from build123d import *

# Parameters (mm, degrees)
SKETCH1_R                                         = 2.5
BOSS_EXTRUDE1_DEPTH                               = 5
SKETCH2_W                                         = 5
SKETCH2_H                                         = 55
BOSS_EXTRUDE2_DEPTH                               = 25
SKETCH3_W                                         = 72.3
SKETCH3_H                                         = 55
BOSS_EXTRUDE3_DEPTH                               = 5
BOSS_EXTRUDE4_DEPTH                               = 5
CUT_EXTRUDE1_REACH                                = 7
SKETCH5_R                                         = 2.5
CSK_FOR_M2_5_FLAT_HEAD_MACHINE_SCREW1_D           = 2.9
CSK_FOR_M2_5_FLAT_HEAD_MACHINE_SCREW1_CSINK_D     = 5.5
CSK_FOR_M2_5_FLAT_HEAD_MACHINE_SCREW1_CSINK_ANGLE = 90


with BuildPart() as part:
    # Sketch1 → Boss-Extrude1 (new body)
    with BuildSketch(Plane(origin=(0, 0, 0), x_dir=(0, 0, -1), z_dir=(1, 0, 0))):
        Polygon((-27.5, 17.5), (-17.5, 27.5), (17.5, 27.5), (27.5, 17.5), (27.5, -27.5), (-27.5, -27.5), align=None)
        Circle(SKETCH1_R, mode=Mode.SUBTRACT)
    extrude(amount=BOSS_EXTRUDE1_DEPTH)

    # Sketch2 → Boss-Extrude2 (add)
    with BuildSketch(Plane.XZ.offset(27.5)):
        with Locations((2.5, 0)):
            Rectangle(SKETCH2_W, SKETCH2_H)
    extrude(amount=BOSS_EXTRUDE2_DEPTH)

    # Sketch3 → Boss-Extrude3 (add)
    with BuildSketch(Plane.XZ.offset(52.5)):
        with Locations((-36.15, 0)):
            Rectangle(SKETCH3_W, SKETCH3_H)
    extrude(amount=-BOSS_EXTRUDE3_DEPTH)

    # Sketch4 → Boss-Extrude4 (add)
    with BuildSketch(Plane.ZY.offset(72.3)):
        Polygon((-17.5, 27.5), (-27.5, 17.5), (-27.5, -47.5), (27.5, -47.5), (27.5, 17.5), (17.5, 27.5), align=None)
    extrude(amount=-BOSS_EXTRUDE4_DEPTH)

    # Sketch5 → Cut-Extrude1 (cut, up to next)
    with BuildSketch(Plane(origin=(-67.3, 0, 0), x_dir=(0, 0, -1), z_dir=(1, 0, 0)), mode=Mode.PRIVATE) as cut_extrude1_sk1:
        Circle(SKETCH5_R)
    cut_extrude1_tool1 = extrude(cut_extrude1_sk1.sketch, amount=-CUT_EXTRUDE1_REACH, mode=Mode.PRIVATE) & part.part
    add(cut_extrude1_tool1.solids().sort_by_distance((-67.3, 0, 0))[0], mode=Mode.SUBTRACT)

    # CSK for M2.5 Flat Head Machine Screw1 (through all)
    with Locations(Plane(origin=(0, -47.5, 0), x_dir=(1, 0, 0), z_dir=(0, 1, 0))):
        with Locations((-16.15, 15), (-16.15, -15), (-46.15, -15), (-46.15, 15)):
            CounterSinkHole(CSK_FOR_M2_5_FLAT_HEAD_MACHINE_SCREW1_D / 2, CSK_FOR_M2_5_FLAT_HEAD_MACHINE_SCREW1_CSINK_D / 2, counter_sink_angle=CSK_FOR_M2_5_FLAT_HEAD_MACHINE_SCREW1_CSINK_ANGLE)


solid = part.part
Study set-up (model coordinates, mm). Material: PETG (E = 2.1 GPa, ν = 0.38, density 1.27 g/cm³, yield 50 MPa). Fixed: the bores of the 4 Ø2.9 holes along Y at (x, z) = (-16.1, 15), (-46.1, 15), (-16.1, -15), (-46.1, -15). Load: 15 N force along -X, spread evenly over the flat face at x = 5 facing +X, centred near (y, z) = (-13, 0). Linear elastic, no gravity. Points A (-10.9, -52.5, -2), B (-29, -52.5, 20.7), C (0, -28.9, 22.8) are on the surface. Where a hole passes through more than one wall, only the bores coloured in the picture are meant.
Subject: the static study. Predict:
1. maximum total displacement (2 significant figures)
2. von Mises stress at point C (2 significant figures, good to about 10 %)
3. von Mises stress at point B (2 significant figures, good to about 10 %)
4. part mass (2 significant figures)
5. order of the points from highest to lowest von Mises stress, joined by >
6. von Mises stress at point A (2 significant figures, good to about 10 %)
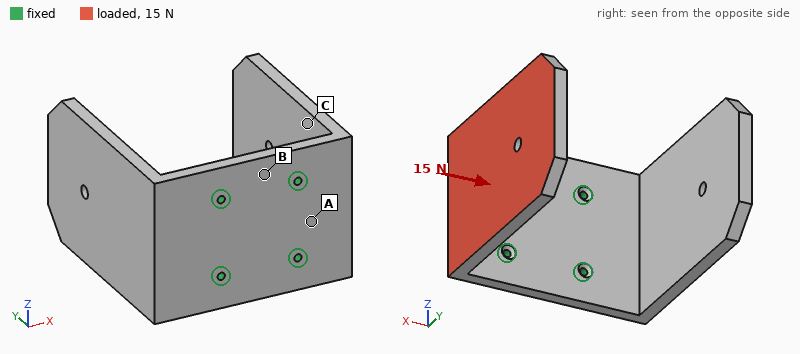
1.3 mm
1.2 MPa
0.44 MPa
78 g
A > C > B
1.8 MPa
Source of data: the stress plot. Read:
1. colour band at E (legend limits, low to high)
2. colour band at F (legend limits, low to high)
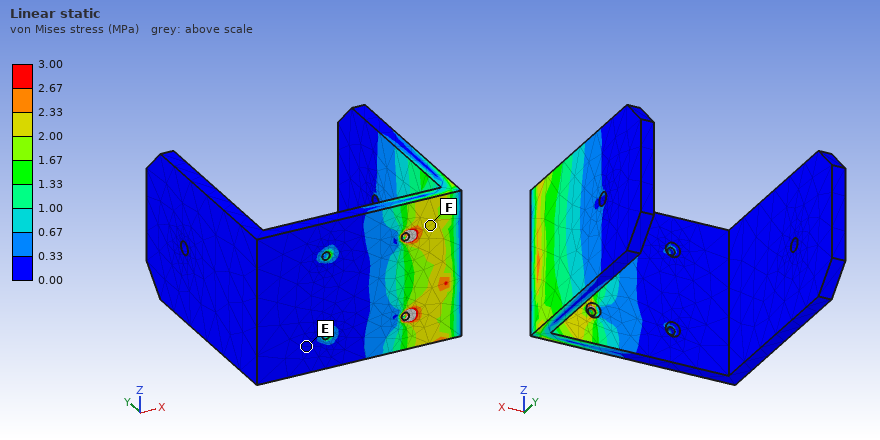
0.00 to 0.33 MPa
2.00 to 2.33 MPa
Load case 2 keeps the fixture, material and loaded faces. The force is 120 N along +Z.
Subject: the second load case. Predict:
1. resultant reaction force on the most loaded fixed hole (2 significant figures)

170 N
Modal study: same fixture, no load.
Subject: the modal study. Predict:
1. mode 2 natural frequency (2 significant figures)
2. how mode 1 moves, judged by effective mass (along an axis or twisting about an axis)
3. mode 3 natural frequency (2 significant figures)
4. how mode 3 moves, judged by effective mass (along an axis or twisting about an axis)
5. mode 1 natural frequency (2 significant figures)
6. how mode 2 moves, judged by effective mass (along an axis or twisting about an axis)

130 Hz
along X
260 Hz
along Z
120 Hz
along X
